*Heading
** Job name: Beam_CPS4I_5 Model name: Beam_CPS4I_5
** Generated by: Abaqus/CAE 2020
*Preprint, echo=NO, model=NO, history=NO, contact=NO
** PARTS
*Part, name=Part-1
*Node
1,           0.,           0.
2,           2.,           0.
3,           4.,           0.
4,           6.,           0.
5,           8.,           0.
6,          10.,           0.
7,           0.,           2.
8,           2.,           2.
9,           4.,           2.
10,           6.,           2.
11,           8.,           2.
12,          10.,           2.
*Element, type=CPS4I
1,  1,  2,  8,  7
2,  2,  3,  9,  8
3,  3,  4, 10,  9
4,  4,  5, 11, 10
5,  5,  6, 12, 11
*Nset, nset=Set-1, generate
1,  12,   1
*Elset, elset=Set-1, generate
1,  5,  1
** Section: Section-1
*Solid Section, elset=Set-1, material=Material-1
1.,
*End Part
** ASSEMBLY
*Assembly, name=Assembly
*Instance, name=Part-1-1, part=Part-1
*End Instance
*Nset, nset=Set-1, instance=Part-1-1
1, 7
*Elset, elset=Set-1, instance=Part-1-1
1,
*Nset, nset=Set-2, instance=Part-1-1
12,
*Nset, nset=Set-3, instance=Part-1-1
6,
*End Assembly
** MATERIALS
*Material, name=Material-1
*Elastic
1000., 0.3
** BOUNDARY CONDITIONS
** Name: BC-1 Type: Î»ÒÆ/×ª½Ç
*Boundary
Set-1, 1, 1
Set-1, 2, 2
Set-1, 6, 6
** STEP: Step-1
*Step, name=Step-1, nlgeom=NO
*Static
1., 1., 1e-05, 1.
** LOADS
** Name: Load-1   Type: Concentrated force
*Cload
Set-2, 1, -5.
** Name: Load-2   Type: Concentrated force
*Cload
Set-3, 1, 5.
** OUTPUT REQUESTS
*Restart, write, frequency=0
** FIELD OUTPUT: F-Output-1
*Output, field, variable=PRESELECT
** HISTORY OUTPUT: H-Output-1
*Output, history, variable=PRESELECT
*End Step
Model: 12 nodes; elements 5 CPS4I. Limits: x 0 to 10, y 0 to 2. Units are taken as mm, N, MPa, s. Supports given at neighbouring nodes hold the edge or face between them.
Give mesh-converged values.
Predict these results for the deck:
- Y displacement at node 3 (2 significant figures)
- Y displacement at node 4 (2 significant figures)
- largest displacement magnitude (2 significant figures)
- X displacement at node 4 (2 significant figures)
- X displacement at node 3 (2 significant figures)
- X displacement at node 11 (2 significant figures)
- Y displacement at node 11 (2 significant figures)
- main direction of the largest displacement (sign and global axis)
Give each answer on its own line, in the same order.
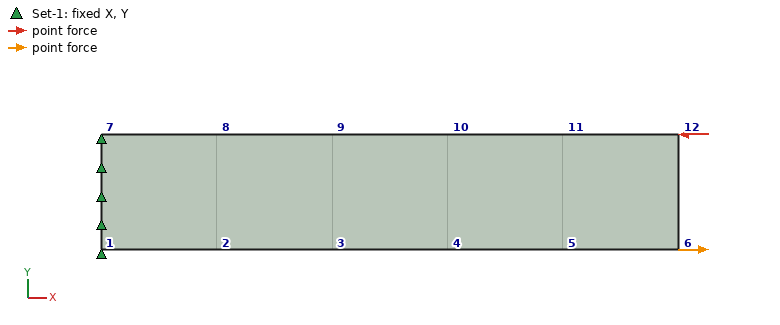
0.12 mm
0.27 mm
0.77 mm
0.089 mm
0.059 mm
-0.12 mm
0.48 mm
+Y
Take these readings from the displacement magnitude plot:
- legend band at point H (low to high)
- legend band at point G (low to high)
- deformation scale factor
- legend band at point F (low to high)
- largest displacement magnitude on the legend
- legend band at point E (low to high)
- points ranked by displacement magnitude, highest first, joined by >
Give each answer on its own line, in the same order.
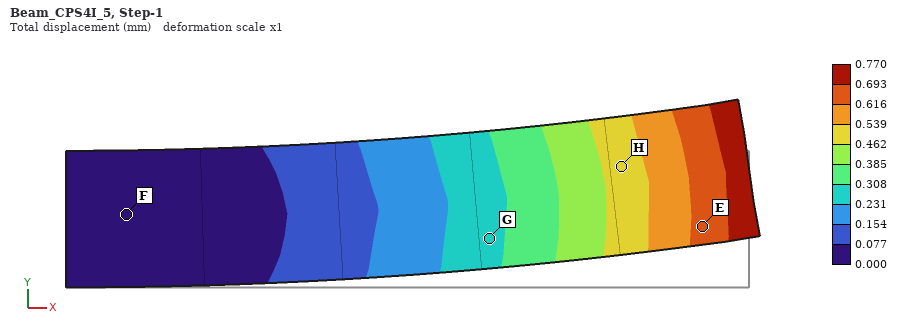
0.462 to 0.539 mm
0.231 to 0.308 mm
1
0.000 to 0.077 mm
0.770 mm
0.616 to 0.693 mm
E > H > G > F
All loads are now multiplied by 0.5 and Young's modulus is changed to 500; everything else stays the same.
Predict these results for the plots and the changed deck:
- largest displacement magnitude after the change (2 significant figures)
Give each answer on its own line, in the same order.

0.77 mm
